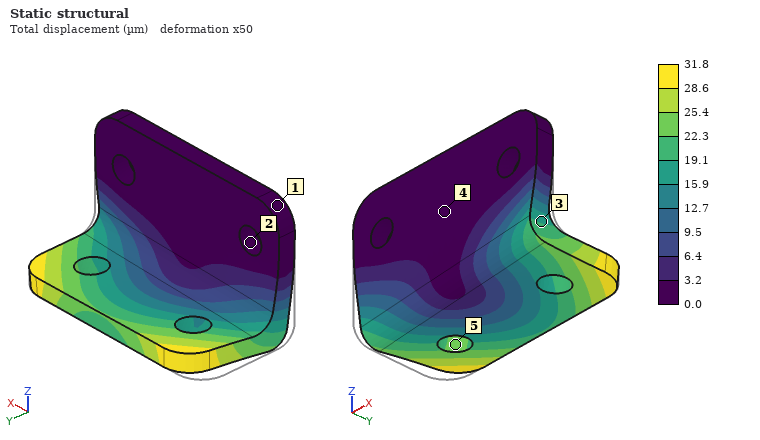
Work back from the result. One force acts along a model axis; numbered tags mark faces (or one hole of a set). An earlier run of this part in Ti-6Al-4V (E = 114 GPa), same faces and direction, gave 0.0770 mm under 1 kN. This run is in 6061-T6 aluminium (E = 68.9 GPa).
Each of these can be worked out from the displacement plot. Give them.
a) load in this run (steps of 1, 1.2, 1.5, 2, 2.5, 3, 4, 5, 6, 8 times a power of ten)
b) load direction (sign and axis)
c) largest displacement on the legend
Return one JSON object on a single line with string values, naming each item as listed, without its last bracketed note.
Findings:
{"load in this run": "250 N", "load direction": "+X", "largest displacement on the legend": "31.8 µm"}
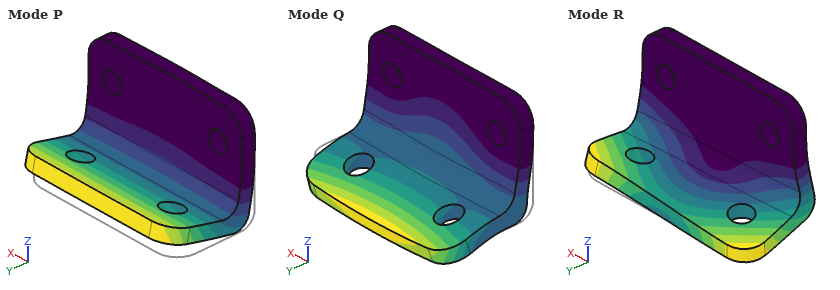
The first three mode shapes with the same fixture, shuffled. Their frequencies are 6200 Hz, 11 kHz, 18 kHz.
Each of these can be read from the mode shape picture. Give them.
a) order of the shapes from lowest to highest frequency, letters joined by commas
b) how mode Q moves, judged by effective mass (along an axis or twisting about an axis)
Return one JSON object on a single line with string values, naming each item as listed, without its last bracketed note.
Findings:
{"order of the shapes from lowest to highest frequency, letters joined by commas": "P, R, Q", "how mode Q moves, judged by effective mass": "along Y"}
